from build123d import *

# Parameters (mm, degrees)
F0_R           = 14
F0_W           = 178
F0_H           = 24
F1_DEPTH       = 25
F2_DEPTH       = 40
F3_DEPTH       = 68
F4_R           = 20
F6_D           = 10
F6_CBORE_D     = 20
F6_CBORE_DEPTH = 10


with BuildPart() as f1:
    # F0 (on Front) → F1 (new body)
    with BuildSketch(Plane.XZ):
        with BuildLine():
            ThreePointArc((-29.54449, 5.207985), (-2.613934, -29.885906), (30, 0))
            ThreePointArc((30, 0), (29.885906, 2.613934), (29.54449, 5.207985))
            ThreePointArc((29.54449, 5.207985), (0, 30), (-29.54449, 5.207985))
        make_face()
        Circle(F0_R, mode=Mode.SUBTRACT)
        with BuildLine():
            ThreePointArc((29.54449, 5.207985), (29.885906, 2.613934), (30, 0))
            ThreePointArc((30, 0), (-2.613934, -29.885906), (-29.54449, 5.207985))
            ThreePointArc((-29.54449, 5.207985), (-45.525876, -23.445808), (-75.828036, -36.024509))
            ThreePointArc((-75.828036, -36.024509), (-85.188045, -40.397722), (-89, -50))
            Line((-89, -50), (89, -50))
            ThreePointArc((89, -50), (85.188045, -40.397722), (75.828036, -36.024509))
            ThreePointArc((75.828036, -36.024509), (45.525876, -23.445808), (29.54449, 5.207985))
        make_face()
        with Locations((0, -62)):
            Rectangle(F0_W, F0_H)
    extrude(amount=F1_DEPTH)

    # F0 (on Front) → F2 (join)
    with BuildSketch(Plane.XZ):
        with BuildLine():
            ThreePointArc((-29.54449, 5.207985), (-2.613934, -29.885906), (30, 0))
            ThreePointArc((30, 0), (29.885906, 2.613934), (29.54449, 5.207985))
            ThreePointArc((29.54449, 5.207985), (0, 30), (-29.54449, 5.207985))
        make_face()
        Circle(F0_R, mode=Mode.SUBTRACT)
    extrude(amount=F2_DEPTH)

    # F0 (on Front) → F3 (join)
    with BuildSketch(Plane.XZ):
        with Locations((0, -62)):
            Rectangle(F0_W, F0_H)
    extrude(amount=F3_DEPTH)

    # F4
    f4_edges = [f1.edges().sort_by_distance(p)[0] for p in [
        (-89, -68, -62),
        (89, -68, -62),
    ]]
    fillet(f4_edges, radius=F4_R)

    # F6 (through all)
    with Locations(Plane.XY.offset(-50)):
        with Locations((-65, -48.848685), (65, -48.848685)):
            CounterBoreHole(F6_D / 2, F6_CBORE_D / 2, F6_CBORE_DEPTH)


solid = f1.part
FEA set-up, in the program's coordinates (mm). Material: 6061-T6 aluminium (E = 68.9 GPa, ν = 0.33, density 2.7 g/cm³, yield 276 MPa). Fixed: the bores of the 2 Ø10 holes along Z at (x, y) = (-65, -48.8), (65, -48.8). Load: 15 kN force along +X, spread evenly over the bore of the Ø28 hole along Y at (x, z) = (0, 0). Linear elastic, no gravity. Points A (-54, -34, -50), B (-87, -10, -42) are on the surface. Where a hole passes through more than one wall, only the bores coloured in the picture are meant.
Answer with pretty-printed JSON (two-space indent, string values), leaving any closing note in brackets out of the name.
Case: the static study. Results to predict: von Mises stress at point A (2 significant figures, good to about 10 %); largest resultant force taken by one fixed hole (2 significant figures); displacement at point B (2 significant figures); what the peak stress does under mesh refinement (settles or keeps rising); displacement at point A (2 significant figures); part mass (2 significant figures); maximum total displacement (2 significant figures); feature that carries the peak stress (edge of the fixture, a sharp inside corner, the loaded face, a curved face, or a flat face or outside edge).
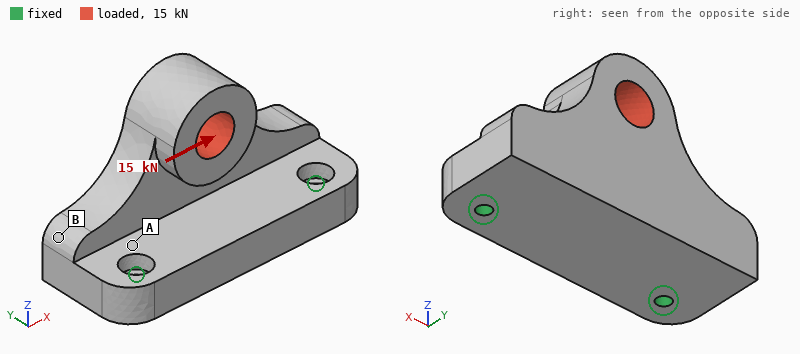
{
  "von Mises stress at point A": "24 MPa",
  "largest resultant force taken by one fixed hole": "11 kN",
  "displacement at point B": "0.059 mm",
  "what the peak stress does under mesh refinement": "keeps rising",
  "displacement at point A": "0.021 mm",
  "part mass": "1.3 kg",
  "maximum total displacement": "0.11 mm",
  "feature that carries the peak stress": "edge of the fixture"
}
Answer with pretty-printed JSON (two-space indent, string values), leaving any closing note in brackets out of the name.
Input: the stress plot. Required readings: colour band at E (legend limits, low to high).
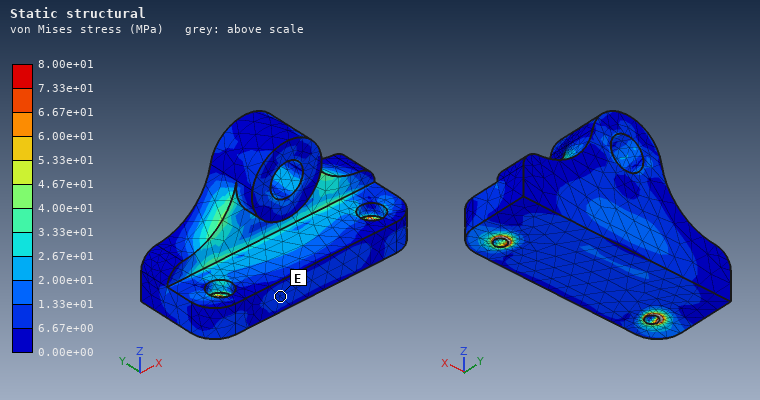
{
  "colour band at E": "6.67e+00 to 1.33e+01 MPa"
}
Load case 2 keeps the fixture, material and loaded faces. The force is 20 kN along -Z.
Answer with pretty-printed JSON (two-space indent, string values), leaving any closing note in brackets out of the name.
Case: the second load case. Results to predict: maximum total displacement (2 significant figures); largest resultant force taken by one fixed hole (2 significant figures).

{
  "maximum total displacement": "0.31 mm",
  "largest resultant force taken by one fixed hole": "10 kN"
}
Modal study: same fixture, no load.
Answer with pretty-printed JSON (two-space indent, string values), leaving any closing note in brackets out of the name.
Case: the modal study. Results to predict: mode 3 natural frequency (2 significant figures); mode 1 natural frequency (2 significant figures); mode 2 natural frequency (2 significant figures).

{
  "mode 3 natural frequency": "3400 Hz",
  "mode 1 natural frequency": "1200 Hz",
  "mode 2 natural frequency": "3300 Hz"
}
